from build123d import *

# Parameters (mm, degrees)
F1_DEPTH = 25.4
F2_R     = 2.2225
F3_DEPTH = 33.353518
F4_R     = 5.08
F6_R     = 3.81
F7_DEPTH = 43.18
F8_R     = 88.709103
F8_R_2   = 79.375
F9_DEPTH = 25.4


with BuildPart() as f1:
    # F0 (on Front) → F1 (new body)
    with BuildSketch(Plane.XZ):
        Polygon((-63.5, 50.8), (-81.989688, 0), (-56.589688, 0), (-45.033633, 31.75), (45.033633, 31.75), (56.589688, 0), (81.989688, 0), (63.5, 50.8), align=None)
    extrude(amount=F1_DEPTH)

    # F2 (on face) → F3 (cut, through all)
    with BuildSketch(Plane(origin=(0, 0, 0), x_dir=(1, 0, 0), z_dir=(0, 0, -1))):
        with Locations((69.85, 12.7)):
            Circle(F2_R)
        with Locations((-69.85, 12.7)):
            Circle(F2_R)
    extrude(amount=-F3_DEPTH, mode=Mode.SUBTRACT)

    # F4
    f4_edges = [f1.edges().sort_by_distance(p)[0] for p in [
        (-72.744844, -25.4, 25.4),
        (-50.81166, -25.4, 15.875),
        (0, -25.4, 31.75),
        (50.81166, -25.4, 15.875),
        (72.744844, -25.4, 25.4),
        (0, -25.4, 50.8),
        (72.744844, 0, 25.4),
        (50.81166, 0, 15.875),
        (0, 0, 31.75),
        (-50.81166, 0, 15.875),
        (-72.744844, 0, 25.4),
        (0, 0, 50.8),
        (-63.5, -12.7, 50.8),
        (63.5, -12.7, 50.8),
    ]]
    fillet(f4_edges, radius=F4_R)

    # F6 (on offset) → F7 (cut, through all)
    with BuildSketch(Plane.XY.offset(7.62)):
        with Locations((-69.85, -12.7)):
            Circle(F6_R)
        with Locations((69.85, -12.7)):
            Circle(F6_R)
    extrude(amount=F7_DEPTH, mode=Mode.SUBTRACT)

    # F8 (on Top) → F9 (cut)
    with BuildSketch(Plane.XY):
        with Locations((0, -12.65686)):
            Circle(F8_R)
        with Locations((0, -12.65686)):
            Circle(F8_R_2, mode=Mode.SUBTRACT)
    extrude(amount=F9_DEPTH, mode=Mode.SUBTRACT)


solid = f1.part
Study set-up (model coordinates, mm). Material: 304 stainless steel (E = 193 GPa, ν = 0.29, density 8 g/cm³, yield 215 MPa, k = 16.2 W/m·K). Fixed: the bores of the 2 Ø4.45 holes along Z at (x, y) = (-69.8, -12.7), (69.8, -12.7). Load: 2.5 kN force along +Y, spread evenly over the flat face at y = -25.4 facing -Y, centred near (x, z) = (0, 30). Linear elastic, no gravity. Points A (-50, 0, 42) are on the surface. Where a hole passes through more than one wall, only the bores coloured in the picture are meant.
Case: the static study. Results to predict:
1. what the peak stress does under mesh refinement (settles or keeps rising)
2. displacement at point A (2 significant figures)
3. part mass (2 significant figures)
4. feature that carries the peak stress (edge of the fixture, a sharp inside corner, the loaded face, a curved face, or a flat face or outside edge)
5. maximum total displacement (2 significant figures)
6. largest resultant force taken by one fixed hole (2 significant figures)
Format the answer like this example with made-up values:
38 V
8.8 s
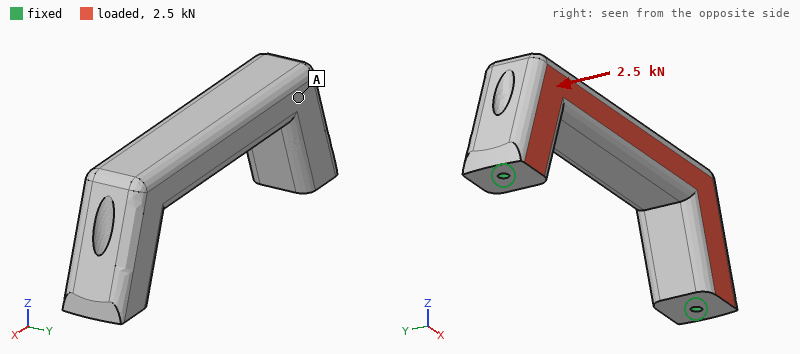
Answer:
keeps rising
36 µm
790 g
edge of the fixture
48 µm
1.3 kN
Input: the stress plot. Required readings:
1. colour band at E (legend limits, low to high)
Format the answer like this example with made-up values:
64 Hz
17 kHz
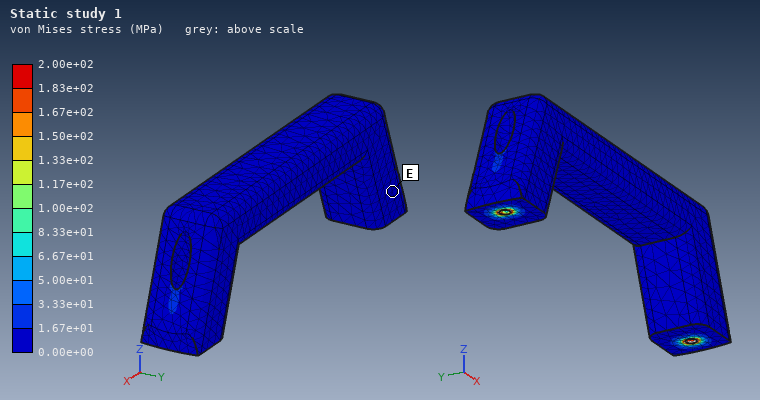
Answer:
0.00e+00 to 1.67e+01 MPa
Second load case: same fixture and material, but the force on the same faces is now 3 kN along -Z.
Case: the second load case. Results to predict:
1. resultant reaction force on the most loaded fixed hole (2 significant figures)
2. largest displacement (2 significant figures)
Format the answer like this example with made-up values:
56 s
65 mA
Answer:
1.7 kN
25 µm
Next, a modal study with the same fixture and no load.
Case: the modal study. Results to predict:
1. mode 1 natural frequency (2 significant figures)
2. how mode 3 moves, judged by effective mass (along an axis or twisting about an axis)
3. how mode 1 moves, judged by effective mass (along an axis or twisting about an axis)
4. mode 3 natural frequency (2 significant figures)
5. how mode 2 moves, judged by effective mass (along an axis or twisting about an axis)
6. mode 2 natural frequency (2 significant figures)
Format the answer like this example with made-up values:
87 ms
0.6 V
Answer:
1500 Hz
twisting about Z
along Y
3700 Hz
along X
3500 Hz
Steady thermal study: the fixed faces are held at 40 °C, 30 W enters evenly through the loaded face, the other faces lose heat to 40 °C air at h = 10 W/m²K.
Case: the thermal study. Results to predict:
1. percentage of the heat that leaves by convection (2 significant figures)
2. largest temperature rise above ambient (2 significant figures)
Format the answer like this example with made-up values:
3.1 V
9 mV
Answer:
24 %
69 K
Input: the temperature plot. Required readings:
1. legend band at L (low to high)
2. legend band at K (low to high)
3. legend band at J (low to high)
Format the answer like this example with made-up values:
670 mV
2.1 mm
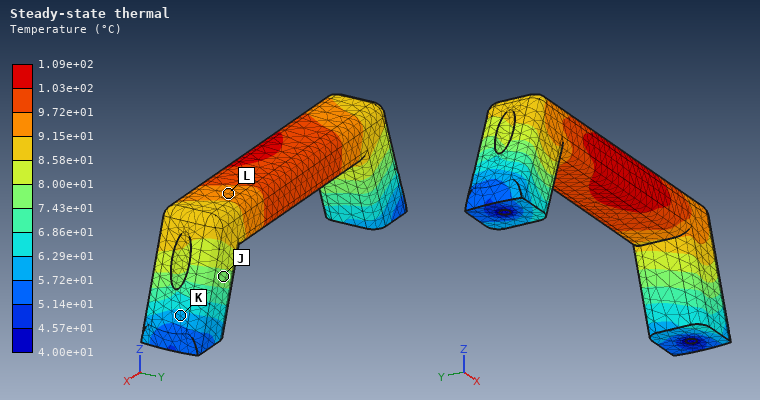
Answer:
9.15e+01 to 9.72e+01 °C
5.72e+01 to 6.29e+01 °C
7.43e+01 to 8.00e+01 °C
